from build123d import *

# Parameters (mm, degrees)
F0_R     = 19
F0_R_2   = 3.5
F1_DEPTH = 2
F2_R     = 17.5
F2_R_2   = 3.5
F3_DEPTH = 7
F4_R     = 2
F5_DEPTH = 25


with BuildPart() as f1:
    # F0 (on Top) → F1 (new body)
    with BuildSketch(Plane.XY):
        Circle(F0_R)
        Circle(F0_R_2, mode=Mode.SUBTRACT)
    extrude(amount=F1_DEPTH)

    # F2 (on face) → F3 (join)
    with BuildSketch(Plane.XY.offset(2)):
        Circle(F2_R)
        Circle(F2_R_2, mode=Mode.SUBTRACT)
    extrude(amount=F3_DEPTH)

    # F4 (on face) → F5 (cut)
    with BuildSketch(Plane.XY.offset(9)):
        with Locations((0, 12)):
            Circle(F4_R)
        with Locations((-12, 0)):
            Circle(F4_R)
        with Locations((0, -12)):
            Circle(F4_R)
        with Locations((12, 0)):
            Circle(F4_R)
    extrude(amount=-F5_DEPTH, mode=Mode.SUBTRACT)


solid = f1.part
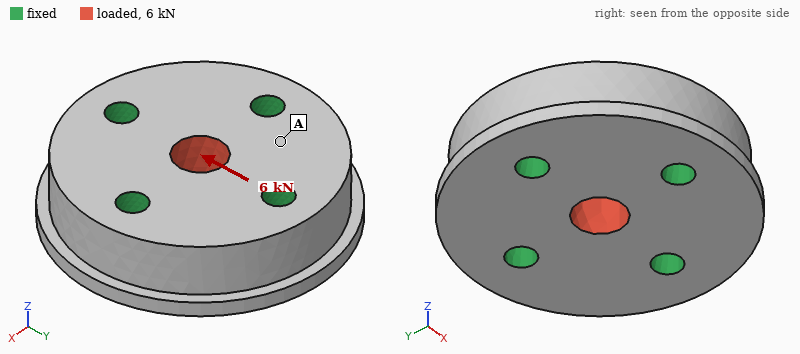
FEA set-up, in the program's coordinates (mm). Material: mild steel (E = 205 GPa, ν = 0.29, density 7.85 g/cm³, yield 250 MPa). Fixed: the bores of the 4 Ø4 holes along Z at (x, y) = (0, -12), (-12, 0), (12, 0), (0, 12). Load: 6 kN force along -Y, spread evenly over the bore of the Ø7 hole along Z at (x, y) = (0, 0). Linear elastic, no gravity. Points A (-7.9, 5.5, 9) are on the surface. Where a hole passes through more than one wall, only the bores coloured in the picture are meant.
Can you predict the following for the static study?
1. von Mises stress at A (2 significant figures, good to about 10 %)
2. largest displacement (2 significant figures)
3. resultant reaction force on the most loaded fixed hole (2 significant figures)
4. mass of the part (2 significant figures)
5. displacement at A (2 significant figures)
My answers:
8.4 MPa
1.3 µm
2.0 kN
64 g
0.44 µm
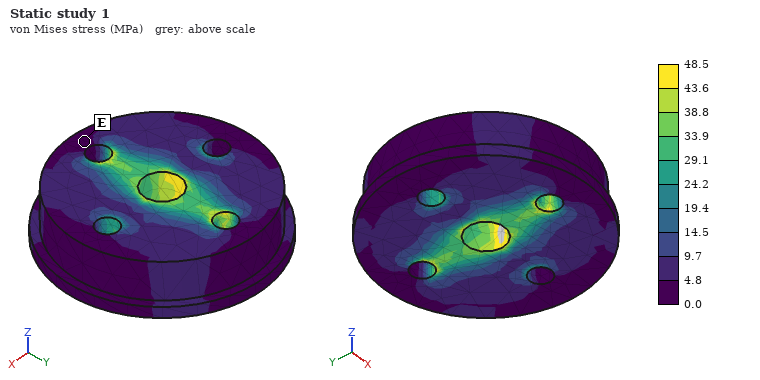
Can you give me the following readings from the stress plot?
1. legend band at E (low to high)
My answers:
0.0 to 4.8 MPa
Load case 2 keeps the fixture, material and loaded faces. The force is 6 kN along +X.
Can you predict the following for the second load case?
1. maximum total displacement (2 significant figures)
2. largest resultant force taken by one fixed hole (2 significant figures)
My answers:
1.3 µm
2.0 kN
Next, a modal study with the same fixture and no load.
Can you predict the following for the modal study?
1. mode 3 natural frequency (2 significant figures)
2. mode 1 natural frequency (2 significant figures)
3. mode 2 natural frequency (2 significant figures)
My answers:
59 kHz
57 kHz
59 kHz
